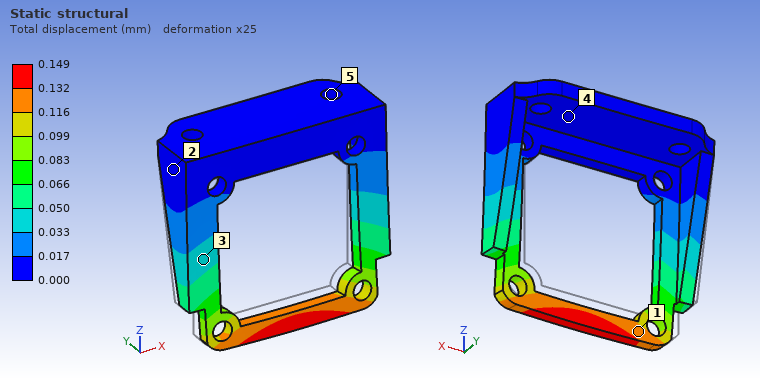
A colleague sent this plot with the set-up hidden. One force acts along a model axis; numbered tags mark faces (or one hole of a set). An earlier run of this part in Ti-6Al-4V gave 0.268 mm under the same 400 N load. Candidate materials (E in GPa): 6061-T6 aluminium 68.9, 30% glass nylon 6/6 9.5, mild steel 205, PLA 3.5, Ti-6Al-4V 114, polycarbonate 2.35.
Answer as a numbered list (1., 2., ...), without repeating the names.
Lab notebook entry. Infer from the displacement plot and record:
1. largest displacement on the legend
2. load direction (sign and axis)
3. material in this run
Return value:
1. 0.149 mm
2. -Y
3. mild steel
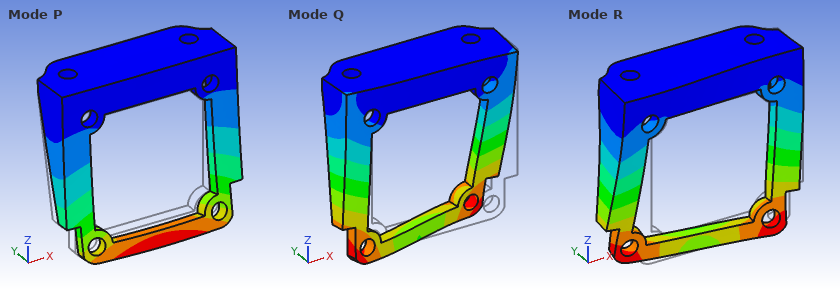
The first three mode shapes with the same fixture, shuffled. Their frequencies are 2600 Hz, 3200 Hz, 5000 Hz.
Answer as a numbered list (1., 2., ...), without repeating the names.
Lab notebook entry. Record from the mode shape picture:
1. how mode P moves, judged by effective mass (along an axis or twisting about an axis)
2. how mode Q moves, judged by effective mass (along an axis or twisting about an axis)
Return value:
1. along Y
2. along X
